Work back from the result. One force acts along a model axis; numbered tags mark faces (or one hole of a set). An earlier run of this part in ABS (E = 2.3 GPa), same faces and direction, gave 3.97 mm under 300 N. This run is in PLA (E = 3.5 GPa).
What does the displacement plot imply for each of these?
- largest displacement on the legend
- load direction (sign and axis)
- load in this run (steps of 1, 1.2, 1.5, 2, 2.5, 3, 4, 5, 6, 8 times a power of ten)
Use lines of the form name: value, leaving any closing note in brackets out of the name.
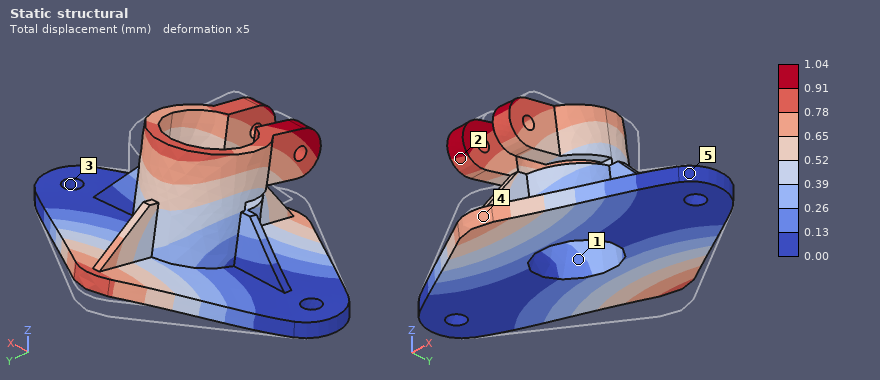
largest displacement on the legend: 1.04 mm
load direction: -Y
load in this run: 120 N
